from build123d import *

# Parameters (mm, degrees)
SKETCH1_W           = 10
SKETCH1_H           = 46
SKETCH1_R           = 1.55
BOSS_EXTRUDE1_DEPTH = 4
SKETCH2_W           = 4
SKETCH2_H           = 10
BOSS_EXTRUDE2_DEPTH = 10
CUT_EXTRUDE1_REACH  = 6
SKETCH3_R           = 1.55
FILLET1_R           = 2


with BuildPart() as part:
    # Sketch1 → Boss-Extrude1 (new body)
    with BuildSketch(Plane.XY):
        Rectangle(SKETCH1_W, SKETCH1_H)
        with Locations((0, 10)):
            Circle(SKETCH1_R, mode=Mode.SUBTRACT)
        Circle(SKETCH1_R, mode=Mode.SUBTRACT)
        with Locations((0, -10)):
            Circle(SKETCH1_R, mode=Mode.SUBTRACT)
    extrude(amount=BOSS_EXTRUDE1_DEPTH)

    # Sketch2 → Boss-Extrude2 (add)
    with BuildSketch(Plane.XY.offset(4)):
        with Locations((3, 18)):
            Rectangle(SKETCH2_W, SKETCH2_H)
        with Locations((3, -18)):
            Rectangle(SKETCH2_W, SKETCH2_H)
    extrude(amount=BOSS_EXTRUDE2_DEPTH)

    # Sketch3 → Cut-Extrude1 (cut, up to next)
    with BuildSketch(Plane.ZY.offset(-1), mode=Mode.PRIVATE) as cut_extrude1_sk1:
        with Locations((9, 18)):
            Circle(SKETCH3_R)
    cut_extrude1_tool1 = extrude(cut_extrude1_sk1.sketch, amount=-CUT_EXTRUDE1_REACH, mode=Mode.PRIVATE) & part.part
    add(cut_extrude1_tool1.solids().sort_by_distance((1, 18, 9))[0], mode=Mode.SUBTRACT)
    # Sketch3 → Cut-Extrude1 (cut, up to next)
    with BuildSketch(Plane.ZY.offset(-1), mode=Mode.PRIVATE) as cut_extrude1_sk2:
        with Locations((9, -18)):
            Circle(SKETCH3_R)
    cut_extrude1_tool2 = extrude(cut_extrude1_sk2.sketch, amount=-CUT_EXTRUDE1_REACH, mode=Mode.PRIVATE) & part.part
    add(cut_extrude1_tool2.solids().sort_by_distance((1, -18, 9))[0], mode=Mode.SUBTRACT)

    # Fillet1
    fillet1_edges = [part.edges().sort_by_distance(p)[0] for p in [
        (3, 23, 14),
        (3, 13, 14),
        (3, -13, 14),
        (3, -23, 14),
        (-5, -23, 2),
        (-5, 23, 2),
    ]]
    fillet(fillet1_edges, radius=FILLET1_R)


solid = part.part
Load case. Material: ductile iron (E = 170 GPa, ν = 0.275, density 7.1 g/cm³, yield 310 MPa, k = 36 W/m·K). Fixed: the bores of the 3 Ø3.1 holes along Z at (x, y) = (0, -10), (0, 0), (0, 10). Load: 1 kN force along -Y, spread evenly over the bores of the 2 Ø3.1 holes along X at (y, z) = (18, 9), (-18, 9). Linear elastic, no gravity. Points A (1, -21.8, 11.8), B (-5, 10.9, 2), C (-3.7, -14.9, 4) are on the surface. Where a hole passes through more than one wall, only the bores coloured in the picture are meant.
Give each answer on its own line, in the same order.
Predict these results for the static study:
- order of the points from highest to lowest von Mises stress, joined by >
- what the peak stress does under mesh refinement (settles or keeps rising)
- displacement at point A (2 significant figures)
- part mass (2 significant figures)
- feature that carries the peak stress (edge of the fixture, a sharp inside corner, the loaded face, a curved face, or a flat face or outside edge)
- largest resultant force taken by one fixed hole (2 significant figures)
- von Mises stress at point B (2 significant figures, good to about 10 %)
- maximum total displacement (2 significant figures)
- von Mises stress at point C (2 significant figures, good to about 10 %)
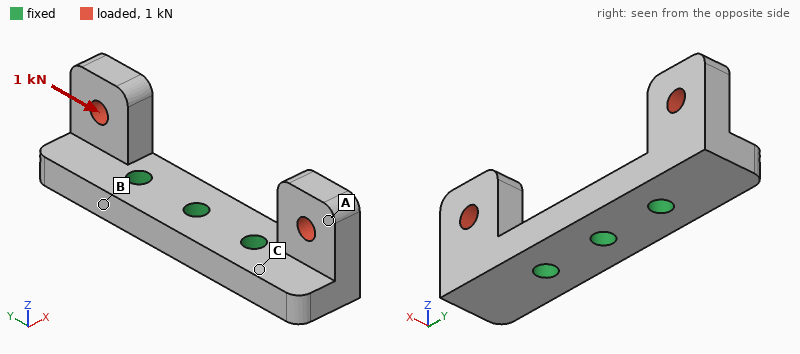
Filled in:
C > B > A
keeps rising
32 µm
18 g
edge of the fixture
460 N
34 MPa
36 µm
71 MPa
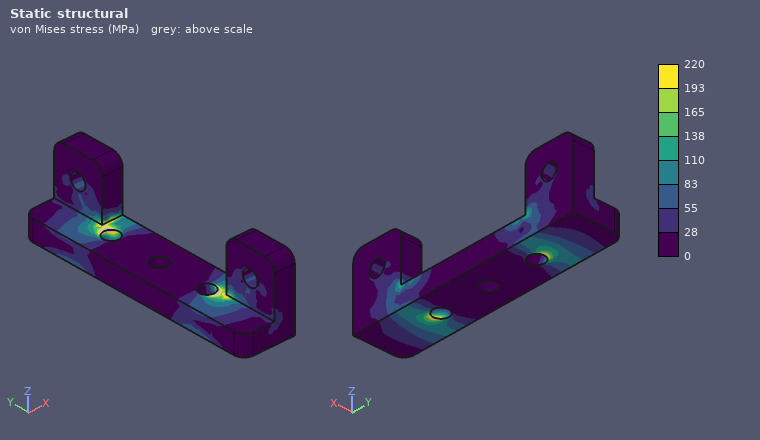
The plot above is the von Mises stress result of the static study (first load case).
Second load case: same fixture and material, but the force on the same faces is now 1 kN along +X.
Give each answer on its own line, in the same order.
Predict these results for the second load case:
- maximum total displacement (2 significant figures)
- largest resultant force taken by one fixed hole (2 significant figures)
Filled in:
42 µm
660 N
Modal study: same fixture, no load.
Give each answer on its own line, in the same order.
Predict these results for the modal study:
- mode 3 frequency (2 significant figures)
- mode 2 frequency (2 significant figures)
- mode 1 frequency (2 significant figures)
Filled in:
13 kHz
11 kHz
11 kHz
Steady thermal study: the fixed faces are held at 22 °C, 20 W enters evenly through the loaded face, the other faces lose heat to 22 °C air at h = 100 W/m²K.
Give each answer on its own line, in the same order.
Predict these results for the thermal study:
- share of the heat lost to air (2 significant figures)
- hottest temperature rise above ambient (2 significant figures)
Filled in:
27 %
80 K
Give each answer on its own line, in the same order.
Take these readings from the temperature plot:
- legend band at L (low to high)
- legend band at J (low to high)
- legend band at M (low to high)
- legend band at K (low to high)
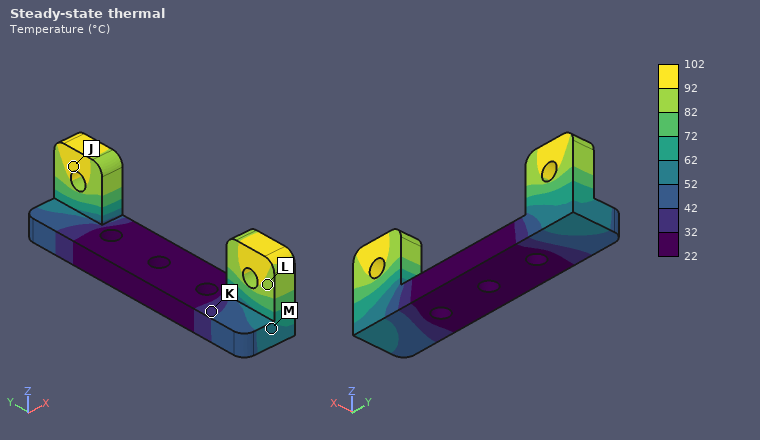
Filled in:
82 to 92 °C
92 to 102 °C
52 to 62 °C
32 to 42 °C
